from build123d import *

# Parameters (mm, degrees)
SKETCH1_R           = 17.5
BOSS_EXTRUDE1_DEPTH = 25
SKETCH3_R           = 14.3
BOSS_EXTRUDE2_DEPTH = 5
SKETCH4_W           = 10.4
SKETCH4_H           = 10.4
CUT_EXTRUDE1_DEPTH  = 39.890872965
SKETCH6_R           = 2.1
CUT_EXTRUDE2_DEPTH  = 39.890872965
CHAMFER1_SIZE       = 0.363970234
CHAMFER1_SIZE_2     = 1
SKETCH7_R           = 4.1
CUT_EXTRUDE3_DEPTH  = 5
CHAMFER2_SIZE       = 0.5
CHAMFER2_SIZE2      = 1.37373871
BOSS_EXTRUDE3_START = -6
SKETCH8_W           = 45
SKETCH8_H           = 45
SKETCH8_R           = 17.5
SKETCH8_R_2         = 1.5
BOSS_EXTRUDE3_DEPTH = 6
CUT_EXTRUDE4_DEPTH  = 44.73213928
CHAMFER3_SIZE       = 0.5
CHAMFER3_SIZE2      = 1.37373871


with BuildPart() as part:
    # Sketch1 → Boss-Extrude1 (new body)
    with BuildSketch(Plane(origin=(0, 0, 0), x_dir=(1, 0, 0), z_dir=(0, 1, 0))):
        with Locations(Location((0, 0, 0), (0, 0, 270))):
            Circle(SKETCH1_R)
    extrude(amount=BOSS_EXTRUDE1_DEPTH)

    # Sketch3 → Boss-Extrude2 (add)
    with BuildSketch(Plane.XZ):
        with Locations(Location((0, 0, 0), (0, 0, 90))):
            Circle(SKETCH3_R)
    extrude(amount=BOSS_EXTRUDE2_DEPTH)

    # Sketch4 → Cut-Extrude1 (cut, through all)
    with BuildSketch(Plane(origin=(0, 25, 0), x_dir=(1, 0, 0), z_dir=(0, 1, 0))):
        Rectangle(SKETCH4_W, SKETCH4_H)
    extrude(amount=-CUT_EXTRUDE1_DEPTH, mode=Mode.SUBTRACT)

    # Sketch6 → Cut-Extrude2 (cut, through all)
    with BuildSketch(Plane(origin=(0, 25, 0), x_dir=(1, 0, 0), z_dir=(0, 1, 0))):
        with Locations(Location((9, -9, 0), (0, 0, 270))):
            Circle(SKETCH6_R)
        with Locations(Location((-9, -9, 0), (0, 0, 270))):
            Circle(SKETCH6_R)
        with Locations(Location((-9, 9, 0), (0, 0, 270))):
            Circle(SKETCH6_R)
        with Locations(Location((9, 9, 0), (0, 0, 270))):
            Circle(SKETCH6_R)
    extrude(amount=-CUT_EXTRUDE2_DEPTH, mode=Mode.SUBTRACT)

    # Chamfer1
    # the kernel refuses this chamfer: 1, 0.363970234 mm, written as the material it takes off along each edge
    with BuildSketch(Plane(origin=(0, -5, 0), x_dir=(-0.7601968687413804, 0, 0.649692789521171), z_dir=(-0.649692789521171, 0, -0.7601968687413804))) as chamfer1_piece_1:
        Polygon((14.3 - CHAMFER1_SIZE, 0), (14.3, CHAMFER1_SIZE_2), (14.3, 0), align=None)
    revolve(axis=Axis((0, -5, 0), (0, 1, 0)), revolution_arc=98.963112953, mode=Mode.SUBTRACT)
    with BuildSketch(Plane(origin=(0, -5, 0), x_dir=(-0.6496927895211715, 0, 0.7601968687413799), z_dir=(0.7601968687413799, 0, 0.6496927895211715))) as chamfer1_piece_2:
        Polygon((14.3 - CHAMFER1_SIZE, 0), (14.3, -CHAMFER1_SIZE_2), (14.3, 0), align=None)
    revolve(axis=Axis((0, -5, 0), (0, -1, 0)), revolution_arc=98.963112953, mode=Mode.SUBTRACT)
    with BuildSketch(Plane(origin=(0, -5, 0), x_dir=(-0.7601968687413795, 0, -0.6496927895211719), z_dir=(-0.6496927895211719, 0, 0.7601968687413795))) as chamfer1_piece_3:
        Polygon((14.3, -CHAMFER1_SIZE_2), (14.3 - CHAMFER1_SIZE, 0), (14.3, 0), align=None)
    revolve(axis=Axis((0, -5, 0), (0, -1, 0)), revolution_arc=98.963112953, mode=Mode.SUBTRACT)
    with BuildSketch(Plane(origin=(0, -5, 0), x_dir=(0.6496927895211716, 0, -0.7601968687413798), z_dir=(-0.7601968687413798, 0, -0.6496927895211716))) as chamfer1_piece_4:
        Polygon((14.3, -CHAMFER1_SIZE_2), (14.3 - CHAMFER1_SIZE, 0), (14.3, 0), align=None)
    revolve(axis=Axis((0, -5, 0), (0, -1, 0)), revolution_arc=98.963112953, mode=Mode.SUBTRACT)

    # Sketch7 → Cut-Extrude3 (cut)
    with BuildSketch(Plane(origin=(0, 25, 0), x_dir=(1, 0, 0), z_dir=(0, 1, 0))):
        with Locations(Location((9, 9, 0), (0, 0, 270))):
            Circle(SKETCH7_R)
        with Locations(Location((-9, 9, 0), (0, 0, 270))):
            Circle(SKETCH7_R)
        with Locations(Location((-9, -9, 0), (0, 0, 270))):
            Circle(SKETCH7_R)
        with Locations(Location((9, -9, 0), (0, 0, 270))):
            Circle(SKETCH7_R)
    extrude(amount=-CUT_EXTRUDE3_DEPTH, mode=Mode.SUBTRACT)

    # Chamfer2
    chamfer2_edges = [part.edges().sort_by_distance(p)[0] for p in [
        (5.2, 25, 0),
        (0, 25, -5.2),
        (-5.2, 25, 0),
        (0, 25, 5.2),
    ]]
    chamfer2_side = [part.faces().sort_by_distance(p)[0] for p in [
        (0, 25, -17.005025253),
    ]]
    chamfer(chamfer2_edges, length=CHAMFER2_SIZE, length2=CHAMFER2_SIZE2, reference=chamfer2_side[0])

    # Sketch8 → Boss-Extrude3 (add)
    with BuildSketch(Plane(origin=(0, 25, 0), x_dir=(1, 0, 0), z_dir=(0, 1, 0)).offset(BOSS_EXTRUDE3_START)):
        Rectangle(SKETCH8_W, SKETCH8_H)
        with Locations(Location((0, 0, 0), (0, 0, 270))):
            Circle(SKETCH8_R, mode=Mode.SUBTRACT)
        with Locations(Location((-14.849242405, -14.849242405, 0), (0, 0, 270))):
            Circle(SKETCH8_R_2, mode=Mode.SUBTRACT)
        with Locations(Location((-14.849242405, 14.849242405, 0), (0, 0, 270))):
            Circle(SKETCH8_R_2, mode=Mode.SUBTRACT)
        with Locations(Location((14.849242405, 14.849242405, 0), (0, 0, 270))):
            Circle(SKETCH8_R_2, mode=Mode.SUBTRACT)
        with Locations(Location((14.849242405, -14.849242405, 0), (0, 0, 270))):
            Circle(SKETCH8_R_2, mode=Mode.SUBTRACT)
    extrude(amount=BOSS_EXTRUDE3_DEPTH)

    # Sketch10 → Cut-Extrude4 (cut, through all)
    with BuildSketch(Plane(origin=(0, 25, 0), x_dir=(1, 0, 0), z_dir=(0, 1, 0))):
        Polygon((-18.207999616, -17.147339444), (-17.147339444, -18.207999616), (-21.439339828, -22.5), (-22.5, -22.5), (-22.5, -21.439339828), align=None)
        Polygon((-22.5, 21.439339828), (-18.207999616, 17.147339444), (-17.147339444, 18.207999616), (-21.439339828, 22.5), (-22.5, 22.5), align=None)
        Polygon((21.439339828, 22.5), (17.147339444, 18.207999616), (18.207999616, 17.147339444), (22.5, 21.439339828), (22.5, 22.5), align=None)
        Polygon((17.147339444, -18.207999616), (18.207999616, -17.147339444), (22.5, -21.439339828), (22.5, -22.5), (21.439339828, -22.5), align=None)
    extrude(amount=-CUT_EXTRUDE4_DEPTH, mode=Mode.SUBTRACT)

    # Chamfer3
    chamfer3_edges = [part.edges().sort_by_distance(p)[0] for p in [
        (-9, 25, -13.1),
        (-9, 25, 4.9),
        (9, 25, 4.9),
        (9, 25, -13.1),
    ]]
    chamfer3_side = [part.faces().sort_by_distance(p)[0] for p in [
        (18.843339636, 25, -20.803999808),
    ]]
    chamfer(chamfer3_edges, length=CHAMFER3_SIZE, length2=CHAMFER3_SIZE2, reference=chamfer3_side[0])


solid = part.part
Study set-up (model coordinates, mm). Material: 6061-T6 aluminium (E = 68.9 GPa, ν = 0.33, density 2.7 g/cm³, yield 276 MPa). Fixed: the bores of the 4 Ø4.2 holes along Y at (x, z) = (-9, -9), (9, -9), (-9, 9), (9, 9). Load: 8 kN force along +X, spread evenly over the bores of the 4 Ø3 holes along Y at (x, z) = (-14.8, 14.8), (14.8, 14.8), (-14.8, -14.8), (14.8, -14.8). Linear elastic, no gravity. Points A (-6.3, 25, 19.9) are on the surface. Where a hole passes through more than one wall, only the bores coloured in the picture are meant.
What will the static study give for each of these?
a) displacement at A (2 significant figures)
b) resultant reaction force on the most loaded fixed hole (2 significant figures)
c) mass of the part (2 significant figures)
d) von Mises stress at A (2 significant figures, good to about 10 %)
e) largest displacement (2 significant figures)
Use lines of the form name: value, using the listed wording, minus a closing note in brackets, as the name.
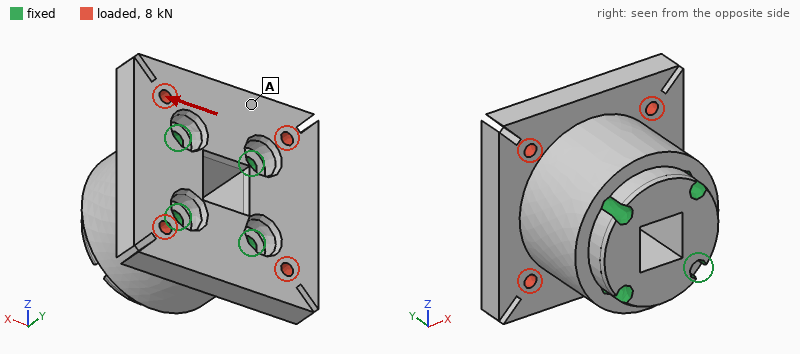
displacement at A: 7.7 µm
resultant reaction force on the most loaded fixed hole: 2.2 kN
mass of the part: 74 g
von Mises stress at A: 14 MPa
largest displacement: 19 µm
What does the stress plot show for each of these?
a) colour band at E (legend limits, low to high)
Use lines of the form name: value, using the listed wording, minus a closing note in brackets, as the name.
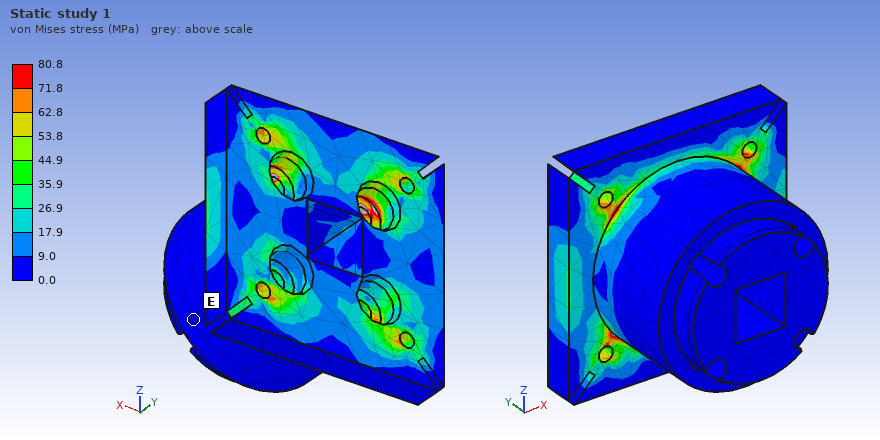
colour band at E: 0.0 to 9.0 MPa
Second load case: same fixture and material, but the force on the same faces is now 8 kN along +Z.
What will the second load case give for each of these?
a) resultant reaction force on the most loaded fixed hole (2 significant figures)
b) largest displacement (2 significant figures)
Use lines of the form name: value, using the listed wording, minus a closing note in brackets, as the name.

resultant reaction force on the most loaded fixed hole: 2.2 kN
largest displacement: 19 µm
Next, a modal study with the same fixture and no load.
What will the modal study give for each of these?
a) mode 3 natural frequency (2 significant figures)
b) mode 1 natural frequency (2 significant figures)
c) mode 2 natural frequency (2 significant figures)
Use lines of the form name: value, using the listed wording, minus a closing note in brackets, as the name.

mode 3 natural frequency: 22 kHz
mode 1 natural frequency: 22 kHz
mode 2 natural frequency: 22 kHz
